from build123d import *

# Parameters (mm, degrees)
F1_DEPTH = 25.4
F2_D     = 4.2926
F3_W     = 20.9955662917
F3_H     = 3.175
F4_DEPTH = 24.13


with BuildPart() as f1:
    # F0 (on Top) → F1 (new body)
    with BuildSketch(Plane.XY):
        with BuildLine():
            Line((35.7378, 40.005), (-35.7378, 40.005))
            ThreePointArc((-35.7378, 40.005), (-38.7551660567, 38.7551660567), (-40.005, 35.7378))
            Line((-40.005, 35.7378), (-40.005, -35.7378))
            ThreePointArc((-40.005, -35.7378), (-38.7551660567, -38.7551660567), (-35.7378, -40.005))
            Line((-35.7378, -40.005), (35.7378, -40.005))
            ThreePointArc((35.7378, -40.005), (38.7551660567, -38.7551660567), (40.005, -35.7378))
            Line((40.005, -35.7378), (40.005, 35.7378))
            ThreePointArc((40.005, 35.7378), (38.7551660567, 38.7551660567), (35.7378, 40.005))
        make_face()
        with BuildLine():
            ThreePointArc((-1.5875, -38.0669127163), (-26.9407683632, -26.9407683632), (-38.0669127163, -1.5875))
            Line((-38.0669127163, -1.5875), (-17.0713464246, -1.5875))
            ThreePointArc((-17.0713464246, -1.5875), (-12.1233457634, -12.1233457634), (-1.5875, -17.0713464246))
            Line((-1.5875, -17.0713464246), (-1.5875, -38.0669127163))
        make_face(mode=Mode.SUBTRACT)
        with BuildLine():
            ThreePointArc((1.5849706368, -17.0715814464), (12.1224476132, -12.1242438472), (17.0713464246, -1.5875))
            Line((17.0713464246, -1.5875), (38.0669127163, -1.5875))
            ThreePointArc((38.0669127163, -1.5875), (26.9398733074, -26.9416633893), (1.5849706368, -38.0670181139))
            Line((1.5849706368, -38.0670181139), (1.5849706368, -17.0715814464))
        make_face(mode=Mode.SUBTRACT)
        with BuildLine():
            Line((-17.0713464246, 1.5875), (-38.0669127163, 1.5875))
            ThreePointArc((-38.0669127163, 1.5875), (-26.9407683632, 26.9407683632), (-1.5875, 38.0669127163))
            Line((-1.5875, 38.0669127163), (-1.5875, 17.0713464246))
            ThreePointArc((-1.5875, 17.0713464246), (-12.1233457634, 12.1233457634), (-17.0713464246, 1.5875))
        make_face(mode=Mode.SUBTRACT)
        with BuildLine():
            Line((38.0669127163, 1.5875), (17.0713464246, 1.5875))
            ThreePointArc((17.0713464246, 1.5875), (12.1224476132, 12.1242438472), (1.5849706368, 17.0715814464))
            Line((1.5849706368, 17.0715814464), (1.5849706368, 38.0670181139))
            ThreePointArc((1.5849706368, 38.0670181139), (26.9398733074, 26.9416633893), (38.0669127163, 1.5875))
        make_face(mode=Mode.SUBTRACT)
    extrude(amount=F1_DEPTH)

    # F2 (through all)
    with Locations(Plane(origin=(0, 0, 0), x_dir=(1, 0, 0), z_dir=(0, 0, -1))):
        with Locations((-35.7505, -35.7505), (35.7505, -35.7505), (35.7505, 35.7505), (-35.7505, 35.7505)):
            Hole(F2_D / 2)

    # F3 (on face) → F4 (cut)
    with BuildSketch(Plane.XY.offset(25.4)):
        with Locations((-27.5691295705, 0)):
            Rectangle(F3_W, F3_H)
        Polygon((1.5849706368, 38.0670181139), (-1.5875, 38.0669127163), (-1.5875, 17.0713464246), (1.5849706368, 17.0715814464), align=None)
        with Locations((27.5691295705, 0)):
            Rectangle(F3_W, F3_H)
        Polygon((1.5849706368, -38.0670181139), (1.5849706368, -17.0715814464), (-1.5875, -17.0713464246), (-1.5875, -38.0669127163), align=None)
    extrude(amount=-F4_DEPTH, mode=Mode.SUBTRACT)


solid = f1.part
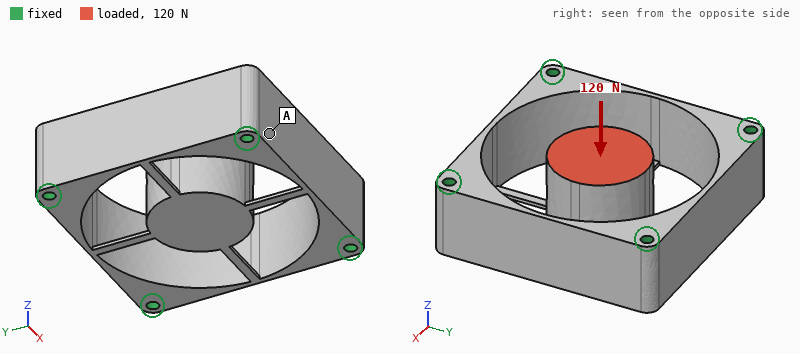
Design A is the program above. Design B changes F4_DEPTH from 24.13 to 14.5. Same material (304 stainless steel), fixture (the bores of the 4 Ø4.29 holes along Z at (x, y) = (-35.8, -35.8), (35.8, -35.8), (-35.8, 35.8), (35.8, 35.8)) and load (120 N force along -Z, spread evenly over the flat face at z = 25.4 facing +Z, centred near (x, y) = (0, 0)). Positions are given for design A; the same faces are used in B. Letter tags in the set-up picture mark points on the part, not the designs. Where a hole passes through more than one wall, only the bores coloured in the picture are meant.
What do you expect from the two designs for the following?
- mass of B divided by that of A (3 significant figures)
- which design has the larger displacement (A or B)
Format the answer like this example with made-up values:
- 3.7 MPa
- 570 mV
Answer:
- 1.04
- A
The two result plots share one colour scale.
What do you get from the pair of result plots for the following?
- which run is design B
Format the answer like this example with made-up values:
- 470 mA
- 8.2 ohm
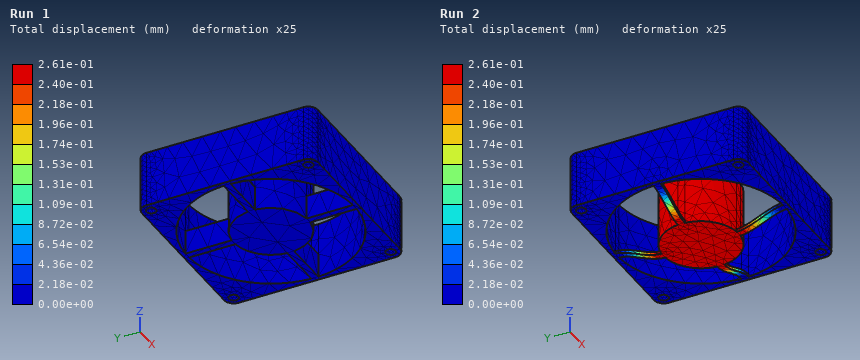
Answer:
- Run 1
